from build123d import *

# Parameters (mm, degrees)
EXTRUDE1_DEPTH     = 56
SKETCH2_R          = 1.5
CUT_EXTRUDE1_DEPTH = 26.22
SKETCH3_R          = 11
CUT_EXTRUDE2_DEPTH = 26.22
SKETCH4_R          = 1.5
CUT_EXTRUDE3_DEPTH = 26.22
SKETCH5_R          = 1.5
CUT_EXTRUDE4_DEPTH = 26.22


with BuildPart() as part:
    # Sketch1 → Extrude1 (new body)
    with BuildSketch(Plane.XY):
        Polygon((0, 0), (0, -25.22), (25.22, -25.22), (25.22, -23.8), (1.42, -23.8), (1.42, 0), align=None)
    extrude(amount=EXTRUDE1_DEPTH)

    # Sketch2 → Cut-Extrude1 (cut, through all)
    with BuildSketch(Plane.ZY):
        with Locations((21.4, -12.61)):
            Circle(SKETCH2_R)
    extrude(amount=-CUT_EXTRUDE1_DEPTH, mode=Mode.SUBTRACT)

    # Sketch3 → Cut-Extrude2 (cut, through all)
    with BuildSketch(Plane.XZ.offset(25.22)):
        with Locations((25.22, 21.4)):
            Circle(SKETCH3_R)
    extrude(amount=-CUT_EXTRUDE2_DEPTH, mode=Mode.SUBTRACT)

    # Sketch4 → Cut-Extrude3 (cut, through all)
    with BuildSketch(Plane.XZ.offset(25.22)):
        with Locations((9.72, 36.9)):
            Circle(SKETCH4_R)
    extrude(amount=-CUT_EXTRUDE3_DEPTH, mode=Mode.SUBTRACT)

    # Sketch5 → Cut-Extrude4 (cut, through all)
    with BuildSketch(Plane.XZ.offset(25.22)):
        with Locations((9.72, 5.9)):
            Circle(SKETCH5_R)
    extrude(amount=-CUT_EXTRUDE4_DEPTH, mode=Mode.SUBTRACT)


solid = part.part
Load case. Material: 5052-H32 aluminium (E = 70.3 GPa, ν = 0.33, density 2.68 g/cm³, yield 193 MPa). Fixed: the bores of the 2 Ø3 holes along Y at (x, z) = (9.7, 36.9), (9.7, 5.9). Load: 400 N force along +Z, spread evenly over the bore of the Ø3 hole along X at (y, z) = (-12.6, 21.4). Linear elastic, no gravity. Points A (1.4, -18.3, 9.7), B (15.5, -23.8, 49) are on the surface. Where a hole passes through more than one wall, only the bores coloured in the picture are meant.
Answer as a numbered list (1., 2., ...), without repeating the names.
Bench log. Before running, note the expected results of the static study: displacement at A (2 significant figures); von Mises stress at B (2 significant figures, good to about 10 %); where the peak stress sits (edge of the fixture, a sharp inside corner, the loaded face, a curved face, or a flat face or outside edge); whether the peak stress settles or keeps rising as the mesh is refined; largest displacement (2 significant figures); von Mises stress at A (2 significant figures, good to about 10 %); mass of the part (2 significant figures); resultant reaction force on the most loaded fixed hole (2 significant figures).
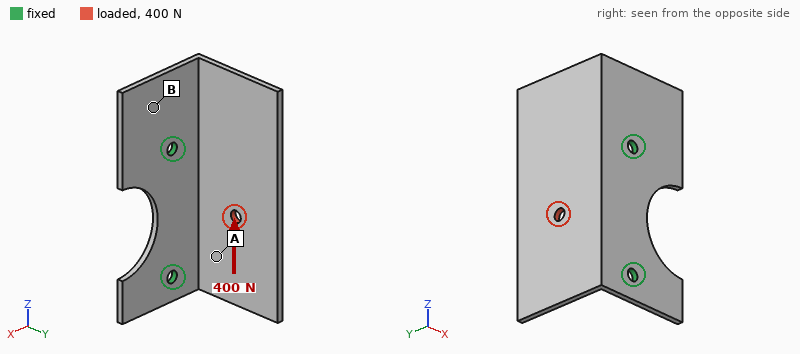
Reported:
1. 0.075 mm
2. 18 MPa
3. edge of the fixture
4. keeps rising
5. 0.27 mm
6. 42 MPa
7. 9.6 g
8. 280 N
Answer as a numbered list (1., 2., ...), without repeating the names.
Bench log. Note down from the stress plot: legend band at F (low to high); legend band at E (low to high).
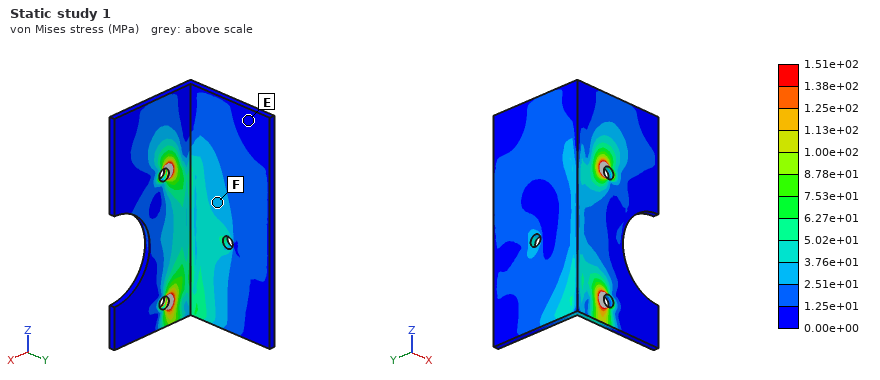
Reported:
1. 2.51e+01 to 3.76e+01 MPa
2. 0.00e+00 to 1.25e+01 MPa
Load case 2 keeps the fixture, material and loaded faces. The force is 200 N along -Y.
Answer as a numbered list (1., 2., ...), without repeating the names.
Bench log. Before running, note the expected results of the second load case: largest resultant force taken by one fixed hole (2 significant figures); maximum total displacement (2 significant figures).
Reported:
1. 100 N
2. 0.29 mm
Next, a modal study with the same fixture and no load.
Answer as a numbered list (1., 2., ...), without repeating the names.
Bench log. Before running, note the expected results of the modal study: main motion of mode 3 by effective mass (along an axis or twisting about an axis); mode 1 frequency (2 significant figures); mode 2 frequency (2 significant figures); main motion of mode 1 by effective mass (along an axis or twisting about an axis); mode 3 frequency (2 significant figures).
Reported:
1. along Y
2. 1200 Hz
3. 2100 Hz
4. along X
5. 3300 Hz
